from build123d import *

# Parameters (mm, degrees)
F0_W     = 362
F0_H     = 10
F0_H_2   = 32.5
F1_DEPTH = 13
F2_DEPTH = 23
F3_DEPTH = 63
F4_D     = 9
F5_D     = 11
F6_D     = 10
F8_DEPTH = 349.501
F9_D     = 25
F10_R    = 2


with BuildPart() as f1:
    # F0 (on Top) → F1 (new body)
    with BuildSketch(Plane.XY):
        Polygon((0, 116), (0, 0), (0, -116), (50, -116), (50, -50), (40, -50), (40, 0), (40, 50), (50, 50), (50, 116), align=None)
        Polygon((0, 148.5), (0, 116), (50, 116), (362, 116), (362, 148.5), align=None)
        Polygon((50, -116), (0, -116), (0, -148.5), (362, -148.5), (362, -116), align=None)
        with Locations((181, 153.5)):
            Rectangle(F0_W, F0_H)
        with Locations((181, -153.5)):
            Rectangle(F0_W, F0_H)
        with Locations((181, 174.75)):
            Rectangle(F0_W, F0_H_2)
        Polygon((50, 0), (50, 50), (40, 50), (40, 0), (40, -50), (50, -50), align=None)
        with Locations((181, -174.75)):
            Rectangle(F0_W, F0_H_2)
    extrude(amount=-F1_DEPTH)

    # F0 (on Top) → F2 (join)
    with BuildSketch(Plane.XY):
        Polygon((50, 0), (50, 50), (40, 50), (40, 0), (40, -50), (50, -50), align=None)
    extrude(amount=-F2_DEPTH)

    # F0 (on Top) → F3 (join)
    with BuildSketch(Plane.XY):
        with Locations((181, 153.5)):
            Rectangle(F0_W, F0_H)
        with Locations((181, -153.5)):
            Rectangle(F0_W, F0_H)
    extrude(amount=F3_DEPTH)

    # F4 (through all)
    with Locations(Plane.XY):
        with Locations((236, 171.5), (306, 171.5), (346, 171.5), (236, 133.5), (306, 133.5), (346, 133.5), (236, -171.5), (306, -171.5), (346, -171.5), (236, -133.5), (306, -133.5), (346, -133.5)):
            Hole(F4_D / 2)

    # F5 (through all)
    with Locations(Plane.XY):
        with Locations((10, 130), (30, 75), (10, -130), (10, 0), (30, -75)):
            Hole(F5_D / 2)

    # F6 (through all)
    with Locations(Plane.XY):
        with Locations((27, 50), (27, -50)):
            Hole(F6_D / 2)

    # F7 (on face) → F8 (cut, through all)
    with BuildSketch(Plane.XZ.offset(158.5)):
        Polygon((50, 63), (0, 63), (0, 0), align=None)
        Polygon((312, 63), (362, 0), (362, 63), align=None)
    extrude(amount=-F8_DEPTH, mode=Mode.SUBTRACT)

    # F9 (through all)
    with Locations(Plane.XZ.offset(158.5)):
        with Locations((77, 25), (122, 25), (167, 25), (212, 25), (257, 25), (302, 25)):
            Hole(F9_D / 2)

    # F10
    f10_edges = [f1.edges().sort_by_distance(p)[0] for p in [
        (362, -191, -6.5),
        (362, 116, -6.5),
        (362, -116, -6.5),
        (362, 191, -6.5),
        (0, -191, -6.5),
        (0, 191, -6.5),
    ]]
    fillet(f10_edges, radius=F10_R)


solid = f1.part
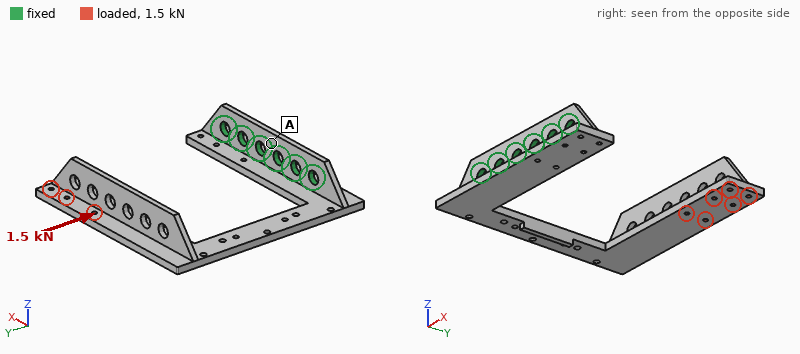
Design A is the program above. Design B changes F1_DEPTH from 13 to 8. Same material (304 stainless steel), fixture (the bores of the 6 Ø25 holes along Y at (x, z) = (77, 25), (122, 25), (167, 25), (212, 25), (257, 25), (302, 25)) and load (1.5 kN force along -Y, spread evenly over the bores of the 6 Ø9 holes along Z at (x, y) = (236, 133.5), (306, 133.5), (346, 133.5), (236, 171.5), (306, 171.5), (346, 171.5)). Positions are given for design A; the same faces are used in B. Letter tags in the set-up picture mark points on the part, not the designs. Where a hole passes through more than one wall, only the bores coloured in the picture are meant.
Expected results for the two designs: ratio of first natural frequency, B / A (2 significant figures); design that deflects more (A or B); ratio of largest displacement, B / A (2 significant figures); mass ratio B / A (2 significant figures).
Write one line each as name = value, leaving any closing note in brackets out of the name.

ratio of first natural frequency, B / A = 0.62
design that deflects more = B
ratio of largest displacement, B / A = 1.6
mass ratio B / A = 0.73
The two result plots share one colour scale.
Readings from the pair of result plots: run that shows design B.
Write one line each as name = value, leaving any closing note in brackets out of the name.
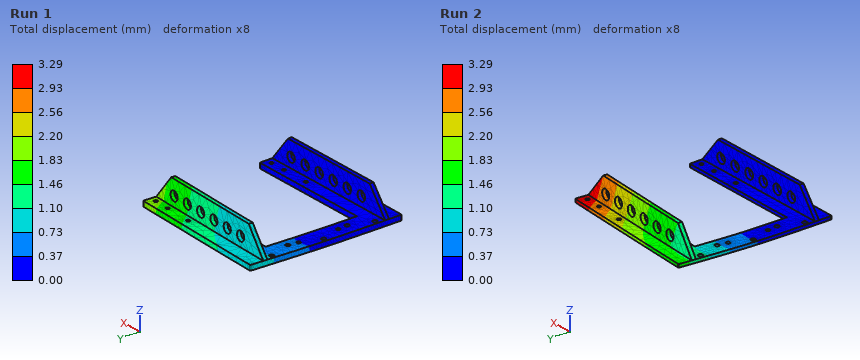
run that shows design B = Run 2
